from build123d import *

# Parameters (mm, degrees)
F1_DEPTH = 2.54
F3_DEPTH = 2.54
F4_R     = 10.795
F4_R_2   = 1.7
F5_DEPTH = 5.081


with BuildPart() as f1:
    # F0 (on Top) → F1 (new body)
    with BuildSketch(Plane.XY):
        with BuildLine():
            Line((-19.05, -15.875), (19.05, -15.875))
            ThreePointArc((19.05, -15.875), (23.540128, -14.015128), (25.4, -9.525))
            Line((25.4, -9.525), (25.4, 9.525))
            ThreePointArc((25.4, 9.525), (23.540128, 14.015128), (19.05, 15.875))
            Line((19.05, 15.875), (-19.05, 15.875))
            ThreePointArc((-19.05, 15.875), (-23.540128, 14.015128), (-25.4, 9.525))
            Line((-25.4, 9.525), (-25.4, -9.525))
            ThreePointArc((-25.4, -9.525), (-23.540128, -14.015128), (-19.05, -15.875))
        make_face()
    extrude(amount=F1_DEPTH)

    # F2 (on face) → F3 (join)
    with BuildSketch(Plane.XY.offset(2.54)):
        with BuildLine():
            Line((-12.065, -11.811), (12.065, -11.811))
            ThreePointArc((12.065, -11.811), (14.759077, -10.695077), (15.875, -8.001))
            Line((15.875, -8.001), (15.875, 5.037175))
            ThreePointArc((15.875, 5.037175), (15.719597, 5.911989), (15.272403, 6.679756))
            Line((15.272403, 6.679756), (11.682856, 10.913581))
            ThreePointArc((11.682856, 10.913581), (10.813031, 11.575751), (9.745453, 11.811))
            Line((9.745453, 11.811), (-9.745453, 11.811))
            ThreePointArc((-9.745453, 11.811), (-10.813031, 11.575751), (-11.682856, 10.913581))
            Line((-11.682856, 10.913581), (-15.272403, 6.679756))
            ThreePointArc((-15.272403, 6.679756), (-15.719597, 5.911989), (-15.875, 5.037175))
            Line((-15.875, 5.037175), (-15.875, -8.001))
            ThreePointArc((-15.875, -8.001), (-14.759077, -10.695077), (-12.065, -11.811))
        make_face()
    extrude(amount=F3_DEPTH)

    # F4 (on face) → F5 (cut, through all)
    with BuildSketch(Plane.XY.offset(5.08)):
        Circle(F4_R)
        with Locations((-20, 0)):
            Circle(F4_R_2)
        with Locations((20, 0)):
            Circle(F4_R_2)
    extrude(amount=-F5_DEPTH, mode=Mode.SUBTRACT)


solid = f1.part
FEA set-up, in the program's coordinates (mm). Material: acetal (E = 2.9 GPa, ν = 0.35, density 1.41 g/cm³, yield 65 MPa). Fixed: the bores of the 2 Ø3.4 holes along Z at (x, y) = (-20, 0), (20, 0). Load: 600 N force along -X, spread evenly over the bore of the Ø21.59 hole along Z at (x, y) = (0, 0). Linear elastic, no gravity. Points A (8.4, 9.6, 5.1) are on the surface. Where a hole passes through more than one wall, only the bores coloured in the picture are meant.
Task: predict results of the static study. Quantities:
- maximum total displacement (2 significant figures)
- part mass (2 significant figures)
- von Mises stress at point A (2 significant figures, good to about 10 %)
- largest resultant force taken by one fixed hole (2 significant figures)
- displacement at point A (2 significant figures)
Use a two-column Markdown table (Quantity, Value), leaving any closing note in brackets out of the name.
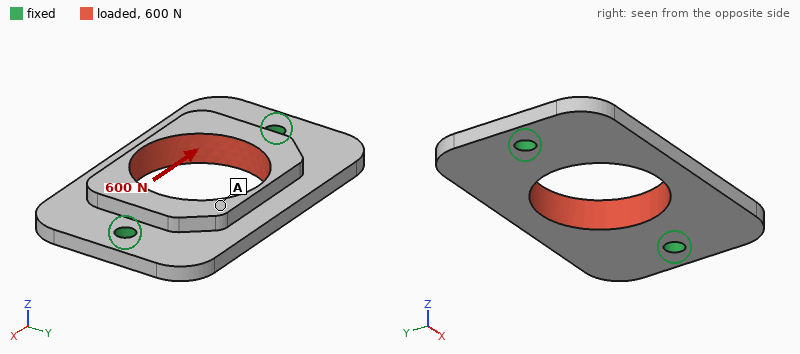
| Quantity | Value |
|---|---|
| maximum total displacement | 66 µm |
| part mass | 5.5 g |
| von Mises stress at point A | 2.2 MPa |
| largest resultant force taken by one fixed hole | 300 N |
| displacement at point A | 59 µm |
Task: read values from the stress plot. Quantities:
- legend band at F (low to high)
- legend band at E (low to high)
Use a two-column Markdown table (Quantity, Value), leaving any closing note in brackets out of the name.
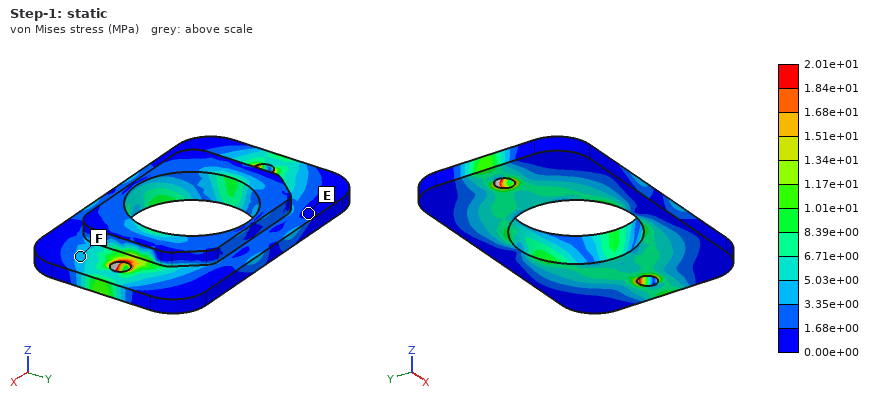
| Quantity | Value |
|---|---|
| legend band at F | 3.35e+00 to 5.03e+00 MPa |
| legend band at E | 0.00e+00 to 1.68e+00 MPa |
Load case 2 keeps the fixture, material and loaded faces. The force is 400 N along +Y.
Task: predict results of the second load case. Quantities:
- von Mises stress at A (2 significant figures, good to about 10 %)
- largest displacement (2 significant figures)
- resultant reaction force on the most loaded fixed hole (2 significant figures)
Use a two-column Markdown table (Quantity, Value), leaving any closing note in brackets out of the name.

| Quantity | Value |
|---|---|
| von Mises stress at A | 2.8 MPa |
| largest displacement | 0.18 mm |
| resultant reaction force on the most loaded fixed hole | 200 N |
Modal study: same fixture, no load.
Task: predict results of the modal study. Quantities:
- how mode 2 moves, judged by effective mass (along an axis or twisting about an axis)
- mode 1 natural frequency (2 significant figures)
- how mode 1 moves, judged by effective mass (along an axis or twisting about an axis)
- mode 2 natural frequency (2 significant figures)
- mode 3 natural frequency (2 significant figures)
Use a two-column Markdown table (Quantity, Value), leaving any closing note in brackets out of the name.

| Quantity | Value |
|---|---|
| how mode 2 moves, judged by effective mass | along Z |
| mode 1 natural frequency | 1700 Hz |
| how mode 1 moves, judged by effective mass | twisting about X |
| mode 2 natural frequency | 2300 Hz |
| mode 3 natural frequency | 3100 Hz |
